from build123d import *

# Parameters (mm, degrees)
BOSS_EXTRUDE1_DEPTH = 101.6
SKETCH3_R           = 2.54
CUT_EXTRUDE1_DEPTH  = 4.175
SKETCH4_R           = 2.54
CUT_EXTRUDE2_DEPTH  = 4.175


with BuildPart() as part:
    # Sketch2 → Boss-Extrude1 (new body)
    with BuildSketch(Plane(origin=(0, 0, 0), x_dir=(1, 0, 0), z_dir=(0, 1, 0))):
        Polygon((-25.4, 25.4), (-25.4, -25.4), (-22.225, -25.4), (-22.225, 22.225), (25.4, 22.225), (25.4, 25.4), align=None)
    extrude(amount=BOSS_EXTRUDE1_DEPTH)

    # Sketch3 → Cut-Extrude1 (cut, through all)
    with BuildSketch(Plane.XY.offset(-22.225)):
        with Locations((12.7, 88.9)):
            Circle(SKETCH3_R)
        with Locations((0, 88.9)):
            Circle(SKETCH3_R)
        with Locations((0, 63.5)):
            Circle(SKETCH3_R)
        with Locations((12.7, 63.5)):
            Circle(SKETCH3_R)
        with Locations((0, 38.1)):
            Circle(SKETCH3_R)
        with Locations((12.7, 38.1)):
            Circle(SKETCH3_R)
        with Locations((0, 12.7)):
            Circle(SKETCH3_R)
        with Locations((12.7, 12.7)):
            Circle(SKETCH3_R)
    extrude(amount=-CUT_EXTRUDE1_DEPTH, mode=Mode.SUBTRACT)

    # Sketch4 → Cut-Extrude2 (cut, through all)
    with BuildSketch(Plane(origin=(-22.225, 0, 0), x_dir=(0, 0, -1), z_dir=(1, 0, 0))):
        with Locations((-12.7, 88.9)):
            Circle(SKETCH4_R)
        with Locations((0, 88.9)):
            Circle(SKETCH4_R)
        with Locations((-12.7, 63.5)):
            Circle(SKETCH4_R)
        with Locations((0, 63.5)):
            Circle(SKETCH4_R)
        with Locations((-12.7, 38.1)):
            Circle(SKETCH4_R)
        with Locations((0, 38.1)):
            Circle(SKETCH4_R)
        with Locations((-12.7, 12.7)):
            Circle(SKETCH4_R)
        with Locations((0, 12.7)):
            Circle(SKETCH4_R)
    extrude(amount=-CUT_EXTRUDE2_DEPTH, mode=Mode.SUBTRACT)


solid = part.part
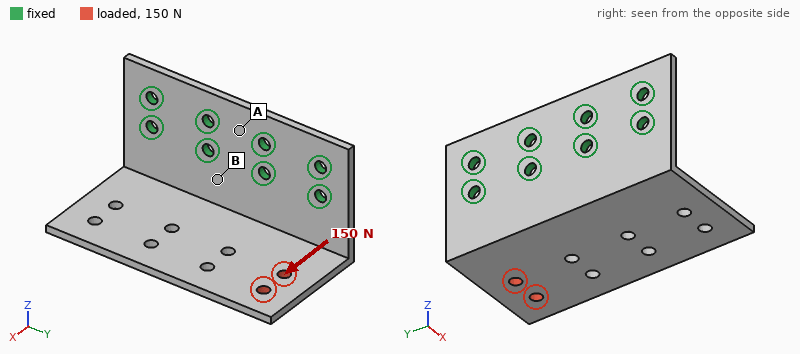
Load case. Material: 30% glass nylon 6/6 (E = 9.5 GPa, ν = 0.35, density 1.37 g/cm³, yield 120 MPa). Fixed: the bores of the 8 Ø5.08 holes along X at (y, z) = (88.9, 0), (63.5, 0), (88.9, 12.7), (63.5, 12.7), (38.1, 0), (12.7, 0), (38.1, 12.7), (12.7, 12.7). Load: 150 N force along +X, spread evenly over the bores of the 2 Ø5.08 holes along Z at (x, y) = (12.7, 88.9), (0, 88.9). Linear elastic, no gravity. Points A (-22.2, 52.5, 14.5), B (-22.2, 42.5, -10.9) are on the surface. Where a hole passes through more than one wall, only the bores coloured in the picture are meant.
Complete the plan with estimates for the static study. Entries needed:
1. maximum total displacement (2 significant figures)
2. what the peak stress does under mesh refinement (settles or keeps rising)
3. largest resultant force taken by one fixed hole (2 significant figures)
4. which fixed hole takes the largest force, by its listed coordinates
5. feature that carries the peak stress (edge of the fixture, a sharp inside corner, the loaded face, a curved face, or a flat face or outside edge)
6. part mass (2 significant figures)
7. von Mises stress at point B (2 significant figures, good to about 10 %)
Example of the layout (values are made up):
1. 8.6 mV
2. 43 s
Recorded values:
1. 1.2 mm
2. keeps rising
3. 140 N
4. (88.9, 0)
5. edge of the fixture
6. 42 g
7. 9.0 MPa
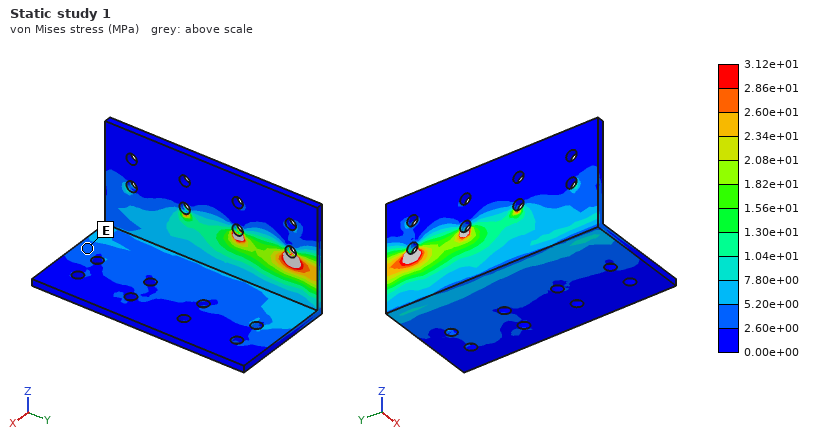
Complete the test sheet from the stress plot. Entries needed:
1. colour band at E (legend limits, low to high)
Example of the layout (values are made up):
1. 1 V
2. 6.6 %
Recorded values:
1. 2.60e+00 to 5.20e+00 MPa
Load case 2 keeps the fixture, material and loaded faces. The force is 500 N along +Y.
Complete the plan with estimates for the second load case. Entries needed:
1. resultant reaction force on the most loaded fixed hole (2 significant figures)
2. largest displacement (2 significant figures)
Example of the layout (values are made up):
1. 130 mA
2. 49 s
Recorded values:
1. 280 N
2. 1.4 mm
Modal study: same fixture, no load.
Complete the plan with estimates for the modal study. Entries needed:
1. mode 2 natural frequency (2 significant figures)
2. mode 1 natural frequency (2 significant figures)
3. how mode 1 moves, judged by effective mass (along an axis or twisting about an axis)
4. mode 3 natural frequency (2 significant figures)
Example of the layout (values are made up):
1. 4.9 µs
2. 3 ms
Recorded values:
1. 600 Hz
2. 340 Hz
3. along Z
4. 1100 Hz
